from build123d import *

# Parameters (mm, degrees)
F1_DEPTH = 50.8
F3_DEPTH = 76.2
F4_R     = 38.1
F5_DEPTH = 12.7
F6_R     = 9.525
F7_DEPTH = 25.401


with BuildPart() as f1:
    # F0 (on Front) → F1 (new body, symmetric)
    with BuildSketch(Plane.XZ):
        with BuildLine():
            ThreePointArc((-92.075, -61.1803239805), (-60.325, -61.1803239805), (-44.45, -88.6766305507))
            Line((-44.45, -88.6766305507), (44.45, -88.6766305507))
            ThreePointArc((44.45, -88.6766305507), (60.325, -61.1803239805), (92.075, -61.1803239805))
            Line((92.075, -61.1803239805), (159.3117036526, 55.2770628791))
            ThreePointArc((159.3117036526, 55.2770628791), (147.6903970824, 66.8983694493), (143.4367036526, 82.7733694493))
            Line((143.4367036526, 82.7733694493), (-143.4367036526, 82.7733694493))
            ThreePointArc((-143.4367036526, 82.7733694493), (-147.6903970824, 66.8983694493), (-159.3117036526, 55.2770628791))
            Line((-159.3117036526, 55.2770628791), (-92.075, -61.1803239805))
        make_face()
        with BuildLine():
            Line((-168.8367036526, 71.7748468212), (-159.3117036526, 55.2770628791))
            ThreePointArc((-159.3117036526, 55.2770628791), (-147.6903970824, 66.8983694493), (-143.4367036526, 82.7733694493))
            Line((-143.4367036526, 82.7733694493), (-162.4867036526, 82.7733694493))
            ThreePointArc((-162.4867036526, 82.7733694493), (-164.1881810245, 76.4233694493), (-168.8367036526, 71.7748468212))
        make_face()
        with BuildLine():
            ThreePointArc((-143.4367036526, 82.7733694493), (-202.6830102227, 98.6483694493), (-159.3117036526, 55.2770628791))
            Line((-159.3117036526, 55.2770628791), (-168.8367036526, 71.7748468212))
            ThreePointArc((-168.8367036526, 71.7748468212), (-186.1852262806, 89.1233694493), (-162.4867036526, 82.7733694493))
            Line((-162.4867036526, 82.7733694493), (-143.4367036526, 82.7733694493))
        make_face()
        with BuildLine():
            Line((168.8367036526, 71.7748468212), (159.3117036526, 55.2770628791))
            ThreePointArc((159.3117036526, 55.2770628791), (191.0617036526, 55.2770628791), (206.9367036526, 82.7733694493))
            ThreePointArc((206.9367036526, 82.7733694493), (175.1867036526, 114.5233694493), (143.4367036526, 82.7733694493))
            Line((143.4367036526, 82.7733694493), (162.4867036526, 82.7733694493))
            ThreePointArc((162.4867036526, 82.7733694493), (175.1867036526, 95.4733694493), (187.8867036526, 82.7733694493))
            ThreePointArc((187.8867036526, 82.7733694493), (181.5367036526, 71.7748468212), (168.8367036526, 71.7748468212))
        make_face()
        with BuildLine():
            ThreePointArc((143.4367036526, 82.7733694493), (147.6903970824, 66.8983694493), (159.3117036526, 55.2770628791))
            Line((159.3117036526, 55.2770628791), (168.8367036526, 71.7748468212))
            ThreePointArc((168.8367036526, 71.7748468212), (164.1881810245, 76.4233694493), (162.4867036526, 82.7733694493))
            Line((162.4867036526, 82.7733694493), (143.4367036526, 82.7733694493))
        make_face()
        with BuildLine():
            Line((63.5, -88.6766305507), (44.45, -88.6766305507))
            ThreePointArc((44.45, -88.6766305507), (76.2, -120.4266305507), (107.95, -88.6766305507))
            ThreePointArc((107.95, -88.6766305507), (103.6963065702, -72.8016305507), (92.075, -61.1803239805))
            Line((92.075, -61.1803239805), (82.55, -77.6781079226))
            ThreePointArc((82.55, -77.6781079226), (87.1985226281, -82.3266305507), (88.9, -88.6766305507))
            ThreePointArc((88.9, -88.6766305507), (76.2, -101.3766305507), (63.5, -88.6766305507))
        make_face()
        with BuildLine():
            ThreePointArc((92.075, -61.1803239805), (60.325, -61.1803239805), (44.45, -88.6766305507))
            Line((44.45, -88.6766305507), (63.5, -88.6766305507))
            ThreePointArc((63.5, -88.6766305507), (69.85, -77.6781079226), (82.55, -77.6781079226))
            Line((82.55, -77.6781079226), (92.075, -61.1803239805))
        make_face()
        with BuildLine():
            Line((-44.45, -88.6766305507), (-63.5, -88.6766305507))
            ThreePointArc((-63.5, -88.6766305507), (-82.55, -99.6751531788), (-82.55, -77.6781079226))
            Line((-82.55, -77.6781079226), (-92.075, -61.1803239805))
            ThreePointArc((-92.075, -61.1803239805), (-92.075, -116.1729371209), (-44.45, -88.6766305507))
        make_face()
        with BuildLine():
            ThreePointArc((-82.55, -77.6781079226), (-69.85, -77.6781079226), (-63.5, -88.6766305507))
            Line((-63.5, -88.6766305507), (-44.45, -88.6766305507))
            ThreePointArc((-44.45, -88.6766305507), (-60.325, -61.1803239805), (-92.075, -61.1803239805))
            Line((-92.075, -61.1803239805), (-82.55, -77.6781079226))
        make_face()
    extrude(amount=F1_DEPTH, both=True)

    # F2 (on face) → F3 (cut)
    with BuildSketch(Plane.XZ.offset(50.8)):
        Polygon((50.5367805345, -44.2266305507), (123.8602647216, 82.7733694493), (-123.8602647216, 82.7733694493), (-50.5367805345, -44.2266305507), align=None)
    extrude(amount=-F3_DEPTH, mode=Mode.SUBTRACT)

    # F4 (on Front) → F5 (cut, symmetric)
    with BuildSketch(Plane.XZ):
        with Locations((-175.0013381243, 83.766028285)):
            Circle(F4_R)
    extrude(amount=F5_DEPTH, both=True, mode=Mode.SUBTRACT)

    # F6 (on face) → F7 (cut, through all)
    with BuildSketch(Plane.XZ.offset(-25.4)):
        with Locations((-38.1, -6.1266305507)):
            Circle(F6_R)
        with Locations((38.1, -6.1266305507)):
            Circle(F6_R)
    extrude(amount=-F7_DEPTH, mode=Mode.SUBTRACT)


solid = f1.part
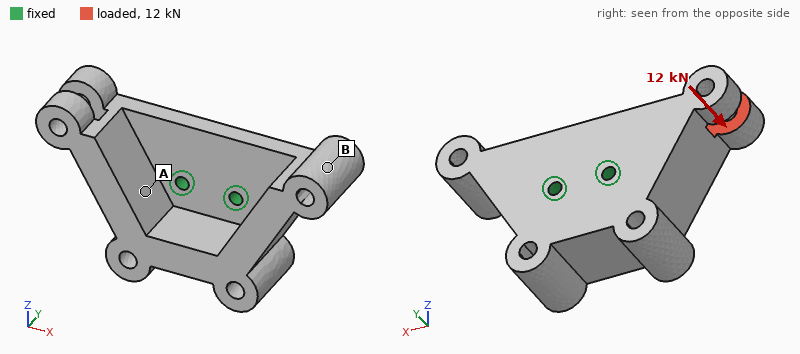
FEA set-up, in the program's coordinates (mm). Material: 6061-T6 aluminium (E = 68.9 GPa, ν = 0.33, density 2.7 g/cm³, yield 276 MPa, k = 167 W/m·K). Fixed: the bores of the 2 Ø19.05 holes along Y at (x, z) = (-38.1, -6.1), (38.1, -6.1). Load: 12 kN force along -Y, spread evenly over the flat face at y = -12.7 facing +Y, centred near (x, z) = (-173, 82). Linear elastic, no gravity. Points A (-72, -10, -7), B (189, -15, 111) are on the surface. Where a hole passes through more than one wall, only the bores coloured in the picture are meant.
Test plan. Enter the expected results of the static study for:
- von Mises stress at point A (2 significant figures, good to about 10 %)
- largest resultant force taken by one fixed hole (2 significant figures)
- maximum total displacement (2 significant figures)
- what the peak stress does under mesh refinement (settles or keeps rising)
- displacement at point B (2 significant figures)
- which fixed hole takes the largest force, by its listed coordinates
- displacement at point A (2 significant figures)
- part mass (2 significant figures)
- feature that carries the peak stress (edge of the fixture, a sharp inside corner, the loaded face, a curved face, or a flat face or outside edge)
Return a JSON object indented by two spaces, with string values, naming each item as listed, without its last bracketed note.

{
  "von Mises stress at point A": "18 MPa",
  "largest resultant force taken by one fixed hole": "25 kN",
  "maximum total displacement": "0.55 mm",
  "what the peak stress does under mesh refinement": "keeps rising",
  "displacement at point B": "0.10 mm",
  "which fixed hole takes the largest force, by its listed coordinates": "(-38.1, -6.1)",
  "displacement at point A": "0.098 mm",
  "part mass": "9.1 kg",
  "feature that carries the peak stress": "edge of the fixture"
}
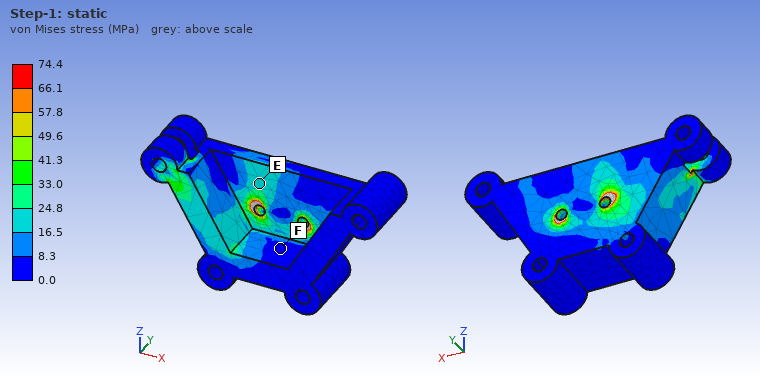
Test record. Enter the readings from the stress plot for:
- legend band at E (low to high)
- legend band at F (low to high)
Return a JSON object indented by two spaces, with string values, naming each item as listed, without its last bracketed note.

{
  "legend band at E": "16.5 to 24.8 MPa",
  "legend band at F": "0.0 to 8.3 MPa"
}
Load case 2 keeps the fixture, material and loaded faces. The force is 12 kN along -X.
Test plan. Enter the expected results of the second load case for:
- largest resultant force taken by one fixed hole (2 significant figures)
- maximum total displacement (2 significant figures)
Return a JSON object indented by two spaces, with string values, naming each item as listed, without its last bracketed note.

{
  "largest resultant force taken by one fixed hole": "14 kN",
  "maximum total displacement": "0.30 mm"
}
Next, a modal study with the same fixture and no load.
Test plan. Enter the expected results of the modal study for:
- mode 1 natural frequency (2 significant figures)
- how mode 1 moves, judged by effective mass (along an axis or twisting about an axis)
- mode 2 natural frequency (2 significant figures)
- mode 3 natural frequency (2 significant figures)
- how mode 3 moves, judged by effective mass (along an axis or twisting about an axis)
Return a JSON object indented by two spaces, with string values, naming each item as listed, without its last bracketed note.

{
  "mode 1 natural frequency": "650 Hz",
  "how mode 1 moves, judged by effective mass": "along Z",
  "mode 2 natural frequency": "800 Hz",
  "mode 3 natural frequency": "1100 Hz",
  "how mode 3 moves, judged by effective mass": "twisting about Y"
}
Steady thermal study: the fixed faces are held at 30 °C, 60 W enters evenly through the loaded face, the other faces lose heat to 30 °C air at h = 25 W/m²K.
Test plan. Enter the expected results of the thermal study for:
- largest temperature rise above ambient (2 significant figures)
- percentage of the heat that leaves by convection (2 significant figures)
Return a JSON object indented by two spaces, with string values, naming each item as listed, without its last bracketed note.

{
  "largest temperature rise above ambient": "22 K",
  "percentage of the heat that leaves by convection": "32 %"
}
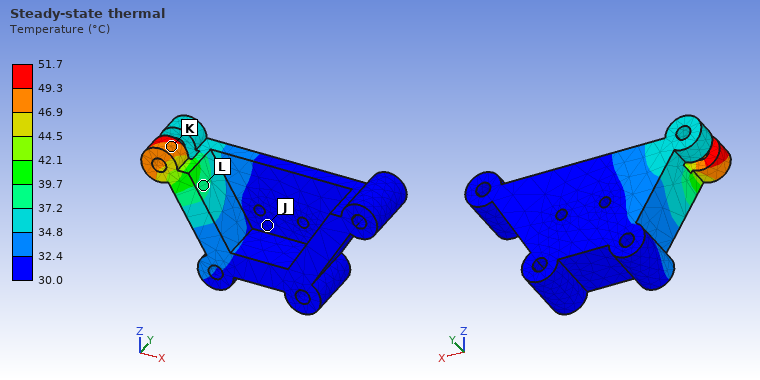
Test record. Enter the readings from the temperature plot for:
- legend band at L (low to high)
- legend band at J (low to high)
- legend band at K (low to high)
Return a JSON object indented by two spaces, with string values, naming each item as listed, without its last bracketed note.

{
  "legend band at L": "37.2 to 39.7 °C",
  "legend band at J": "30.0 to 32.4 °C",
  "legend band at K": "46.9 to 49.3 °C"
}
